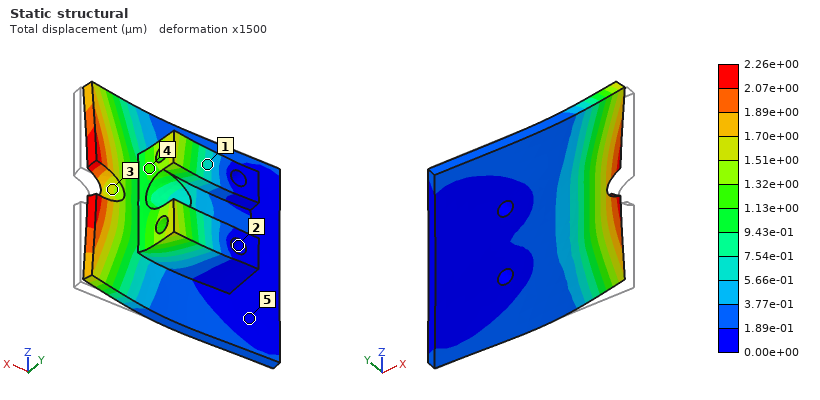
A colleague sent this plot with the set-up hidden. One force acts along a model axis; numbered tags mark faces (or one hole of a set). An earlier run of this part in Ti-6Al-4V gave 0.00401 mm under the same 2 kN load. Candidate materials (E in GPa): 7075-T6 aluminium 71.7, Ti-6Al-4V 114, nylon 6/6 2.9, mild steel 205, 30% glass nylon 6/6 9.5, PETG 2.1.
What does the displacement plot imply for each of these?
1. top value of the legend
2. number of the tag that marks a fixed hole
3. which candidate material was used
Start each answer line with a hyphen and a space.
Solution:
- 2.26e+00 µm
- 2
- mild steel
